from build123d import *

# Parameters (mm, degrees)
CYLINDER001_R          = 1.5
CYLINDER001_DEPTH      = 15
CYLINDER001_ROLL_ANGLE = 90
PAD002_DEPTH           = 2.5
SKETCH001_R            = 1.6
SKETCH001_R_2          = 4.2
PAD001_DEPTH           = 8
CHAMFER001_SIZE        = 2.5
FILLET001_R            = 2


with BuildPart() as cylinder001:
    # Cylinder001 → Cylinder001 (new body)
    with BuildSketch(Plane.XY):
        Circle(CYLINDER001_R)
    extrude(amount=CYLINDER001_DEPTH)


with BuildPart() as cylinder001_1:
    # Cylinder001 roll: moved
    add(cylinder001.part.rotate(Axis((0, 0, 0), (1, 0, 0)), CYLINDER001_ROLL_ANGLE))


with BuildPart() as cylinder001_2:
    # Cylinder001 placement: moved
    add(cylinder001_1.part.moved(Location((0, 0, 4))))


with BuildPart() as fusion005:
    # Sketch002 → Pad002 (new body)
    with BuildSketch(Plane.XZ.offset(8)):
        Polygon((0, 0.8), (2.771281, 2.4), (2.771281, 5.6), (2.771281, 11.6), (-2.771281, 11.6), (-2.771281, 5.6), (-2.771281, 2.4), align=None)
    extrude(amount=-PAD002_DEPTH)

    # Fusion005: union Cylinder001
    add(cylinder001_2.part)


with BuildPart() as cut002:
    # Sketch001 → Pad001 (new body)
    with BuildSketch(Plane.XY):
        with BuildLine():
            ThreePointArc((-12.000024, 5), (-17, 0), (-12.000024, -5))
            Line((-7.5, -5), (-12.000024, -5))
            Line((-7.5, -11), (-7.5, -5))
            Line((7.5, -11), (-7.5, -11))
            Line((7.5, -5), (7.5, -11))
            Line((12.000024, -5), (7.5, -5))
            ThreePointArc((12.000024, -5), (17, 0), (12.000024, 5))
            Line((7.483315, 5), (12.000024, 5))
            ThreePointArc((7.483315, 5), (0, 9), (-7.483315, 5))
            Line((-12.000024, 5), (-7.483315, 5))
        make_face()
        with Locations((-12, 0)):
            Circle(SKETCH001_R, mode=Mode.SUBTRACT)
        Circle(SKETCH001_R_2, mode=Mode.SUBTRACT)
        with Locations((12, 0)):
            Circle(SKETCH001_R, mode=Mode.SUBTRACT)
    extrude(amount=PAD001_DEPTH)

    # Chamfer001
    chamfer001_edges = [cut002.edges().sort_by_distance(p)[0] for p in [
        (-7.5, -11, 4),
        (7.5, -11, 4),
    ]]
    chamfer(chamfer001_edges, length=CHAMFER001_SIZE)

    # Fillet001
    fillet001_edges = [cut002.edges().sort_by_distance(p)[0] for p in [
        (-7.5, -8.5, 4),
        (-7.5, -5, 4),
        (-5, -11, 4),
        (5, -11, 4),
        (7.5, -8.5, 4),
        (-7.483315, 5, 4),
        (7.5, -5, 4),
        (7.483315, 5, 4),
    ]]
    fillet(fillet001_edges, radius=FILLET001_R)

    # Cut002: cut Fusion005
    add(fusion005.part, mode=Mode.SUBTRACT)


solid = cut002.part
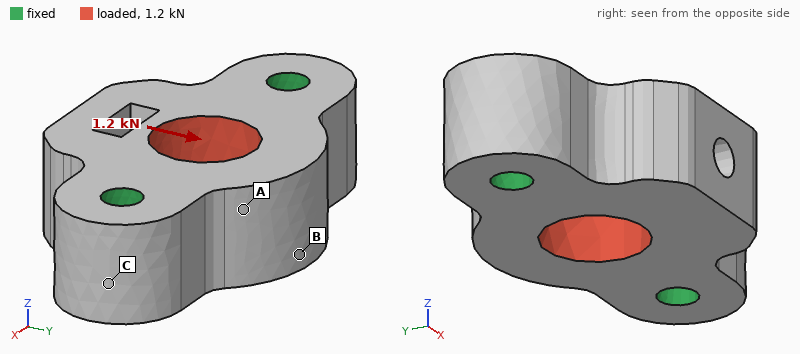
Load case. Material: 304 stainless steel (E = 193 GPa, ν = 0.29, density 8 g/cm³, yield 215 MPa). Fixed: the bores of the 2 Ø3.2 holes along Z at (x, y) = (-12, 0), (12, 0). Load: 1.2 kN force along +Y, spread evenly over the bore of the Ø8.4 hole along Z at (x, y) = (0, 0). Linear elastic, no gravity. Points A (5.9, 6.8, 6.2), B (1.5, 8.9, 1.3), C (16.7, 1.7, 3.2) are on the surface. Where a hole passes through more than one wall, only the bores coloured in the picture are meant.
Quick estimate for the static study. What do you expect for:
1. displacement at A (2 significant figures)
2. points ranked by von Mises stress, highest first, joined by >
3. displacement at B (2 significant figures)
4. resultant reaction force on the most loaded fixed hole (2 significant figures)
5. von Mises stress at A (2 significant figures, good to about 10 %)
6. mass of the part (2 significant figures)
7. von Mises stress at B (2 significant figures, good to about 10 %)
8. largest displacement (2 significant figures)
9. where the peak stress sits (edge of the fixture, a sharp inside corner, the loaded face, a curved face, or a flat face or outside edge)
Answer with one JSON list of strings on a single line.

["0.88 µm", "A > B > C", "1.1 µm", "600 N", "12 MPa", "23 g", "8.9 MPa", "1.5 µm", "a curved face"]
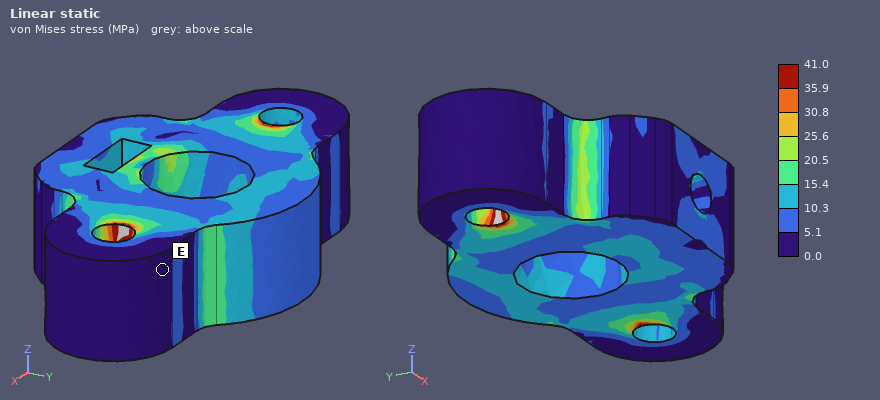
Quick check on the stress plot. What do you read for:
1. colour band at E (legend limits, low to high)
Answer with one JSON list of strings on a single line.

["0.0 to 5.1 MPa"]
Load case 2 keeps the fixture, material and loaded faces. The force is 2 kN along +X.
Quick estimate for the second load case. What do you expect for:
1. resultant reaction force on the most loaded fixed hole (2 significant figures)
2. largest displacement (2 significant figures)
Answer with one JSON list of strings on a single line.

["1.0 kN", "0.85 µm"]
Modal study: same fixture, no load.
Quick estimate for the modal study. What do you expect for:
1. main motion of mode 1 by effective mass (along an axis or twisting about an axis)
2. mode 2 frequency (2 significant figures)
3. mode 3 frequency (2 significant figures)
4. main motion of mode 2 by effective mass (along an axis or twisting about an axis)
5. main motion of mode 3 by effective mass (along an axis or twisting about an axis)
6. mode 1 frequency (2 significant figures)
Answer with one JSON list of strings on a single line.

["along Z", "38 kHz", "50 kHz", "along Z", "along Y", "30 kHz"]
